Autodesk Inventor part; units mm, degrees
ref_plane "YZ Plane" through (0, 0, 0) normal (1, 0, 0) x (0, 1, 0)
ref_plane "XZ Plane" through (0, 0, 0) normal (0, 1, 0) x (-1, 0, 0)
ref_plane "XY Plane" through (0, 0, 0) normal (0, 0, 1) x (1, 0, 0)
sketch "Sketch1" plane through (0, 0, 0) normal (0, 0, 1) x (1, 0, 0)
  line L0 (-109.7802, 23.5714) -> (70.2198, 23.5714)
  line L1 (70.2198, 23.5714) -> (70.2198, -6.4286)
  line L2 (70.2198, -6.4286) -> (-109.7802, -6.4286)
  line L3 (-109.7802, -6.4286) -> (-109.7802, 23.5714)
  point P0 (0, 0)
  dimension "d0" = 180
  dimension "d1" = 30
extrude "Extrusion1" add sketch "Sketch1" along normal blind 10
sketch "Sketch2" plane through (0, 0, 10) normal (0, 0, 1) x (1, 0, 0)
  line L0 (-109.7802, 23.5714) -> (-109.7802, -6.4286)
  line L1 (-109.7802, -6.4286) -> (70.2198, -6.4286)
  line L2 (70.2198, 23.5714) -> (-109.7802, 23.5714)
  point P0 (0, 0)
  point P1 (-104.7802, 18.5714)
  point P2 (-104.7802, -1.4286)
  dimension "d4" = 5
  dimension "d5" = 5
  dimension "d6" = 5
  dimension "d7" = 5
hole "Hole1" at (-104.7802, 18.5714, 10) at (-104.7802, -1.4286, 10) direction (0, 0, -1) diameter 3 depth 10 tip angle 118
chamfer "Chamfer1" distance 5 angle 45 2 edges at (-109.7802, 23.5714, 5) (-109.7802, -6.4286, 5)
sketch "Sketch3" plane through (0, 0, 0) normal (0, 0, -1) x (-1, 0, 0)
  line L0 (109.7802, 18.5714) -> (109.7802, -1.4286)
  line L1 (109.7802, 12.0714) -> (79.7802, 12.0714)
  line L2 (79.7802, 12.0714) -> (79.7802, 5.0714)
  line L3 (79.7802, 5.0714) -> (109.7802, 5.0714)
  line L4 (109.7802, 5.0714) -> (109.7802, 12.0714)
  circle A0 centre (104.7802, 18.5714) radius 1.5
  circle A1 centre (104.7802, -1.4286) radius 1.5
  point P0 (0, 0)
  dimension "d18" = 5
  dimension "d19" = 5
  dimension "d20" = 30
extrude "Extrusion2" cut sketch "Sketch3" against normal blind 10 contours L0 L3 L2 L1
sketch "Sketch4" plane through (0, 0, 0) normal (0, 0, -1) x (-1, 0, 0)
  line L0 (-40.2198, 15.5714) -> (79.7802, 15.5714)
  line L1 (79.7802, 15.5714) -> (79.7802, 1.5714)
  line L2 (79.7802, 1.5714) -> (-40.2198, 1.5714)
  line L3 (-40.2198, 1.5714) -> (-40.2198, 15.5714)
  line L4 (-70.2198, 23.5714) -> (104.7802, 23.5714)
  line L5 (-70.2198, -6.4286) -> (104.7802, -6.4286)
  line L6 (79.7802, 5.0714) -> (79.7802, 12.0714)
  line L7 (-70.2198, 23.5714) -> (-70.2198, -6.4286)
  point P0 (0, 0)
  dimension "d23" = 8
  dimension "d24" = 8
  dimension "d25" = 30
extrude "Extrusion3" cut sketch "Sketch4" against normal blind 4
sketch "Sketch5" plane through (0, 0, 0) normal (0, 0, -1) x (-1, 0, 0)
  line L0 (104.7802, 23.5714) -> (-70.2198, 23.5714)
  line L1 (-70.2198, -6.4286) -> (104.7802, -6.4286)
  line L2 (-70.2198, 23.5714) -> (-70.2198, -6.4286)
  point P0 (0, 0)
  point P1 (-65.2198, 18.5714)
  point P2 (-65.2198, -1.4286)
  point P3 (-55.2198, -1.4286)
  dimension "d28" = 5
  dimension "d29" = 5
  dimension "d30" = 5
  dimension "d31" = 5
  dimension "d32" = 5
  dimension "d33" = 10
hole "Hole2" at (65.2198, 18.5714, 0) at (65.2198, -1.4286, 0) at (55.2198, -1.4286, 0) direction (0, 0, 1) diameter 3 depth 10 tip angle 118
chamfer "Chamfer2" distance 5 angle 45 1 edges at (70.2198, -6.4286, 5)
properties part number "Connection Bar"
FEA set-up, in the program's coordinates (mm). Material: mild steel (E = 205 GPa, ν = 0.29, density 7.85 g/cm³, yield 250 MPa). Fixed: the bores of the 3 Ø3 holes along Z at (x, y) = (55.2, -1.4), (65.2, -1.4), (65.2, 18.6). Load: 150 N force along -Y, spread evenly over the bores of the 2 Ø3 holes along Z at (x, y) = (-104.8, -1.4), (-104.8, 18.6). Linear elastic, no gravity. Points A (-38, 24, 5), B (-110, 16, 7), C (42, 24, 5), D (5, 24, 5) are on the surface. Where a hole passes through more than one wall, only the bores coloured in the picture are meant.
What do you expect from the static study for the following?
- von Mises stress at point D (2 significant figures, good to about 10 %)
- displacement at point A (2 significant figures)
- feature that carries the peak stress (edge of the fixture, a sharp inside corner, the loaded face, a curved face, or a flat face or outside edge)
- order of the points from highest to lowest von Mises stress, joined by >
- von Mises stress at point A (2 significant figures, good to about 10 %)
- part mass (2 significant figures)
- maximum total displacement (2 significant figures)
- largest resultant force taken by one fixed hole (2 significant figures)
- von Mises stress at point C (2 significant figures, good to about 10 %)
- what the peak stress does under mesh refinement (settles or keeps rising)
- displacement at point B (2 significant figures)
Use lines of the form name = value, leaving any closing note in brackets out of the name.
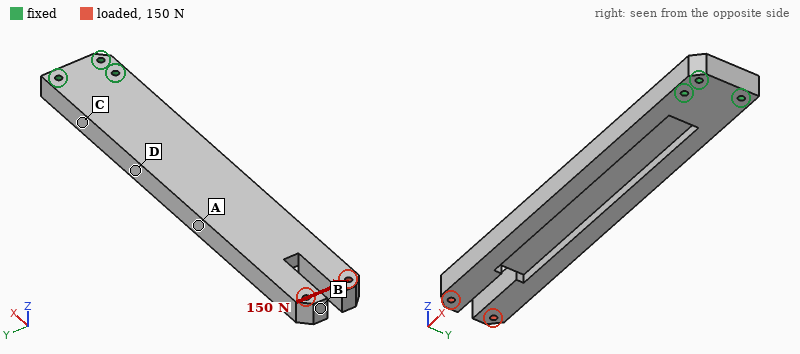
von Mises stress at point D = 11 MPa
displacement at point A = 24 µm
feature that carries the peak stress = edge of the fixture
order of the points from highest to lowest von Mises stress, joined by > = C > D > A > B
von Mises stress at point A = 7.1 MPa
part mass = 350 g
maximum total displacement = 60 µm
largest resultant force taken by one fixed hole = 1.0 kN
von Mises stress at point C = 16 MPa
what the peak stress does under mesh refinement = keeps rising
displacement at point B = 59 µm
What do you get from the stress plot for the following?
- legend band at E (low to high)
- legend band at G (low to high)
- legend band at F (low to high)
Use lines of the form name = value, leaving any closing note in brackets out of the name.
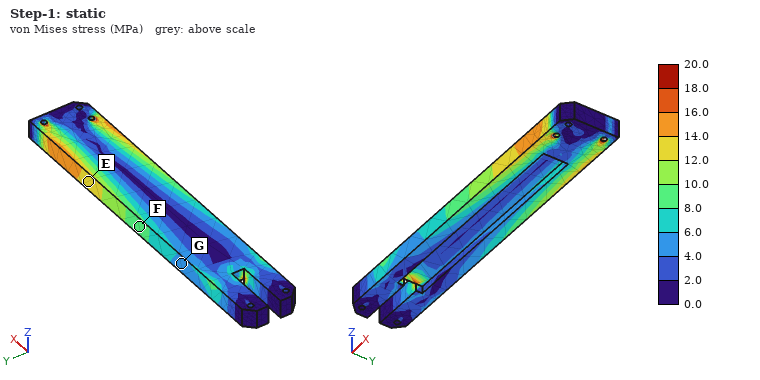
legend band at E = 12.0 to 14.0 MPa
legend band at G = 4.0 to 6.0 MPa
legend band at F = 8.0 to 10.0 MPa
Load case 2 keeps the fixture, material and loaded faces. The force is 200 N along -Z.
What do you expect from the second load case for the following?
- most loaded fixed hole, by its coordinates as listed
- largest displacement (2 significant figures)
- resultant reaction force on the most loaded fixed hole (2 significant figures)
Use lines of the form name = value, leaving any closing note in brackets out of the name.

most loaded fixed hole, by its coordinates as listed = (55.2, -1.4)
largest displacement = 0.78 mm
resultant reaction force on the most loaded fixed hole = 1.0 kN
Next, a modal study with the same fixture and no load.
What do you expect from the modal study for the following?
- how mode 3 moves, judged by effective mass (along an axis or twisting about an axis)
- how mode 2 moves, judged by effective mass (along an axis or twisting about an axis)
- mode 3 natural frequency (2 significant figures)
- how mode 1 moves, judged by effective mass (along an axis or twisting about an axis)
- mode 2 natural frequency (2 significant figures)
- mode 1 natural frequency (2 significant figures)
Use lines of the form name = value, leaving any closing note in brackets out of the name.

how mode 3 moves, judged by effective mass = along Z
how mode 2 moves, judged by effective mass = along Y
mode 3 natural frequency = 1800 Hz
how mode 1 moves, judged by effective mass = along Z
mode 2 natural frequency = 920 Hz
mode 1 natural frequency = 290 Hz
